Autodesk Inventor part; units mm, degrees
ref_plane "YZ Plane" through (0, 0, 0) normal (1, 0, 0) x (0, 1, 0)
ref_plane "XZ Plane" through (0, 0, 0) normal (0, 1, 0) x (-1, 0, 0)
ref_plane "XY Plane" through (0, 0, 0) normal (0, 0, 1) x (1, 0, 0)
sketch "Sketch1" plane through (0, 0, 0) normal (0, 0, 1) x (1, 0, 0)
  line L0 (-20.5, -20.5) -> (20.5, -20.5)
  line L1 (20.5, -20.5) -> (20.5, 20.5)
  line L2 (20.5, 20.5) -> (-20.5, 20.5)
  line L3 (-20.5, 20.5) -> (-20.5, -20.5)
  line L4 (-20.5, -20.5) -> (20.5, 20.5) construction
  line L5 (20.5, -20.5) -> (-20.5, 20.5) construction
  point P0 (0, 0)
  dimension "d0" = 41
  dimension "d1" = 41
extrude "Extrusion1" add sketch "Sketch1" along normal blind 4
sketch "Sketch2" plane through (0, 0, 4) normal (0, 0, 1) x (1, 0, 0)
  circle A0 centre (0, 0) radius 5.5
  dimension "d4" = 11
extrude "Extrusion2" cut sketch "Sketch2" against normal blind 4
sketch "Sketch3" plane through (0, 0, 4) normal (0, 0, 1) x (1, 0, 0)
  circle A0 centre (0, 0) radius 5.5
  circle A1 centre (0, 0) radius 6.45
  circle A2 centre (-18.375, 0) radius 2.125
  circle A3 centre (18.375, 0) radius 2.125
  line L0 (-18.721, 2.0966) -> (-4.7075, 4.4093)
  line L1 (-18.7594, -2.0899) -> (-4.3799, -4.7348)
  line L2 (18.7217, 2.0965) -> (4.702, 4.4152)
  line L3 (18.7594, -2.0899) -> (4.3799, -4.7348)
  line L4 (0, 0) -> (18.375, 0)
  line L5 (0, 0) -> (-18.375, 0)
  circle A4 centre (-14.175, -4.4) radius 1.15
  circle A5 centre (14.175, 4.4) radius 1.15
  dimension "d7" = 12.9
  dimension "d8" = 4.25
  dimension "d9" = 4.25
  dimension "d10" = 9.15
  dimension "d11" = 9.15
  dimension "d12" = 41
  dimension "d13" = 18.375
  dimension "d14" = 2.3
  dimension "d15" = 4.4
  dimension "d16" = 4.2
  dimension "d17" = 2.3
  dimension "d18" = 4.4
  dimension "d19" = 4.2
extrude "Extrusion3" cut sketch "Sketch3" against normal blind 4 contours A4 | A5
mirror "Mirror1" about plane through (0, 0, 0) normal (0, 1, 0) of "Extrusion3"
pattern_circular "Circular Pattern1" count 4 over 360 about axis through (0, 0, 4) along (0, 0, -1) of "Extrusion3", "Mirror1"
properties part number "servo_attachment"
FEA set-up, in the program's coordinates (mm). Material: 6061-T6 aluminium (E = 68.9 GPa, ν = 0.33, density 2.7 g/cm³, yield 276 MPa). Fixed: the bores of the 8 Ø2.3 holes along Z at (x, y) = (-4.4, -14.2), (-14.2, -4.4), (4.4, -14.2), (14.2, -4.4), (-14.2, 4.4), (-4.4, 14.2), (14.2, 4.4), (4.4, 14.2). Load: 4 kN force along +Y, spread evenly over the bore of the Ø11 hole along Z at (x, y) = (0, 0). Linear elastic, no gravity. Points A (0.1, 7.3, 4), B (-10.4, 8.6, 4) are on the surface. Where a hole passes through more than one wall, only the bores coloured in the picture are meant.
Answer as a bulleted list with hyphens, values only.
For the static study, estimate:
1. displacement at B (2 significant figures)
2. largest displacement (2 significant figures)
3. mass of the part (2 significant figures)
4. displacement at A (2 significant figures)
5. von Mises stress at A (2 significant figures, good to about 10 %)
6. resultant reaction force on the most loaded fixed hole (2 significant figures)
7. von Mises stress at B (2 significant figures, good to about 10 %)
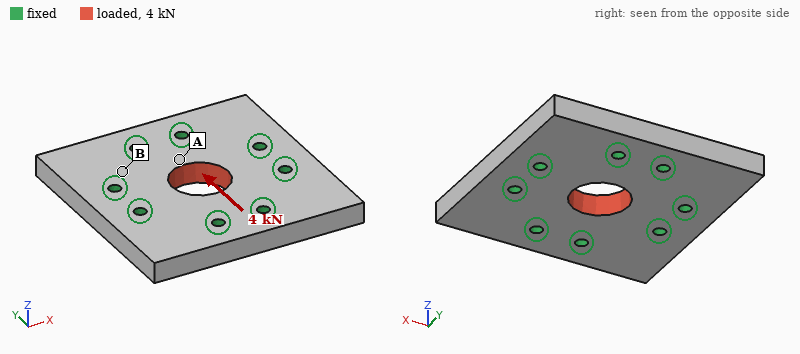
- 1.2 µm
- 4.2 µm
- 17 g
- 2.9 µm
- 27 MPa
- 740 N
- 7.9 MPa
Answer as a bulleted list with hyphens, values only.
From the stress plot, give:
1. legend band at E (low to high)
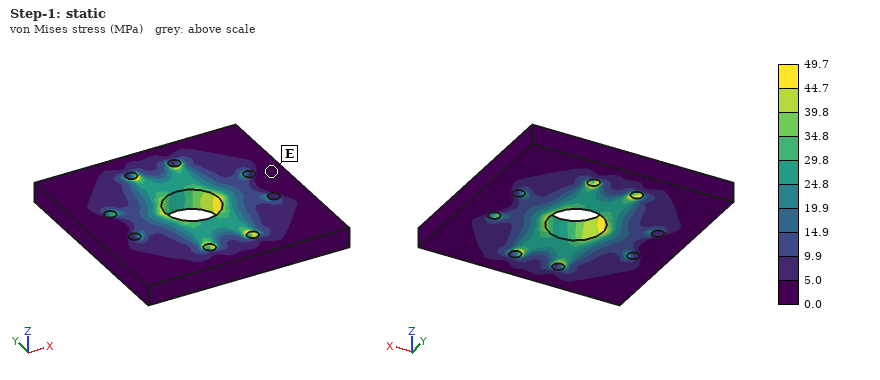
- 0.0 to 5.0 MPa
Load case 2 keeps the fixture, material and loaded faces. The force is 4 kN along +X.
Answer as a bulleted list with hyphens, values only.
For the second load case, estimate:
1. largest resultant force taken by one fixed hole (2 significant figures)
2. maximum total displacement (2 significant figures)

- 740 N
- 4.2 µm
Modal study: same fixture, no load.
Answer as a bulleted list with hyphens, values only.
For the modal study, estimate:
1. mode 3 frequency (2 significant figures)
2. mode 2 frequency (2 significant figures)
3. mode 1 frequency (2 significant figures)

- 20 kHz
- 20 kHz
- 20 kHz
